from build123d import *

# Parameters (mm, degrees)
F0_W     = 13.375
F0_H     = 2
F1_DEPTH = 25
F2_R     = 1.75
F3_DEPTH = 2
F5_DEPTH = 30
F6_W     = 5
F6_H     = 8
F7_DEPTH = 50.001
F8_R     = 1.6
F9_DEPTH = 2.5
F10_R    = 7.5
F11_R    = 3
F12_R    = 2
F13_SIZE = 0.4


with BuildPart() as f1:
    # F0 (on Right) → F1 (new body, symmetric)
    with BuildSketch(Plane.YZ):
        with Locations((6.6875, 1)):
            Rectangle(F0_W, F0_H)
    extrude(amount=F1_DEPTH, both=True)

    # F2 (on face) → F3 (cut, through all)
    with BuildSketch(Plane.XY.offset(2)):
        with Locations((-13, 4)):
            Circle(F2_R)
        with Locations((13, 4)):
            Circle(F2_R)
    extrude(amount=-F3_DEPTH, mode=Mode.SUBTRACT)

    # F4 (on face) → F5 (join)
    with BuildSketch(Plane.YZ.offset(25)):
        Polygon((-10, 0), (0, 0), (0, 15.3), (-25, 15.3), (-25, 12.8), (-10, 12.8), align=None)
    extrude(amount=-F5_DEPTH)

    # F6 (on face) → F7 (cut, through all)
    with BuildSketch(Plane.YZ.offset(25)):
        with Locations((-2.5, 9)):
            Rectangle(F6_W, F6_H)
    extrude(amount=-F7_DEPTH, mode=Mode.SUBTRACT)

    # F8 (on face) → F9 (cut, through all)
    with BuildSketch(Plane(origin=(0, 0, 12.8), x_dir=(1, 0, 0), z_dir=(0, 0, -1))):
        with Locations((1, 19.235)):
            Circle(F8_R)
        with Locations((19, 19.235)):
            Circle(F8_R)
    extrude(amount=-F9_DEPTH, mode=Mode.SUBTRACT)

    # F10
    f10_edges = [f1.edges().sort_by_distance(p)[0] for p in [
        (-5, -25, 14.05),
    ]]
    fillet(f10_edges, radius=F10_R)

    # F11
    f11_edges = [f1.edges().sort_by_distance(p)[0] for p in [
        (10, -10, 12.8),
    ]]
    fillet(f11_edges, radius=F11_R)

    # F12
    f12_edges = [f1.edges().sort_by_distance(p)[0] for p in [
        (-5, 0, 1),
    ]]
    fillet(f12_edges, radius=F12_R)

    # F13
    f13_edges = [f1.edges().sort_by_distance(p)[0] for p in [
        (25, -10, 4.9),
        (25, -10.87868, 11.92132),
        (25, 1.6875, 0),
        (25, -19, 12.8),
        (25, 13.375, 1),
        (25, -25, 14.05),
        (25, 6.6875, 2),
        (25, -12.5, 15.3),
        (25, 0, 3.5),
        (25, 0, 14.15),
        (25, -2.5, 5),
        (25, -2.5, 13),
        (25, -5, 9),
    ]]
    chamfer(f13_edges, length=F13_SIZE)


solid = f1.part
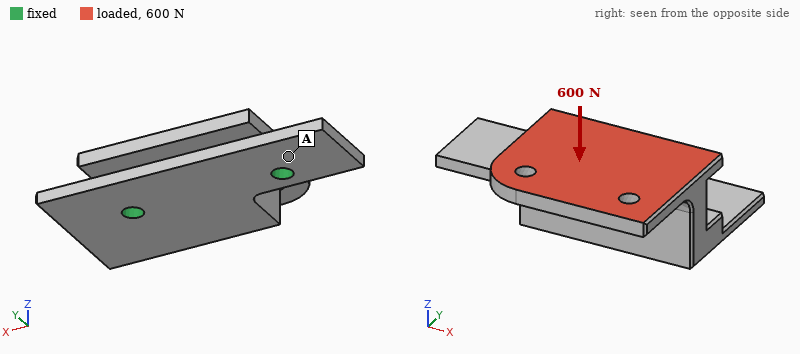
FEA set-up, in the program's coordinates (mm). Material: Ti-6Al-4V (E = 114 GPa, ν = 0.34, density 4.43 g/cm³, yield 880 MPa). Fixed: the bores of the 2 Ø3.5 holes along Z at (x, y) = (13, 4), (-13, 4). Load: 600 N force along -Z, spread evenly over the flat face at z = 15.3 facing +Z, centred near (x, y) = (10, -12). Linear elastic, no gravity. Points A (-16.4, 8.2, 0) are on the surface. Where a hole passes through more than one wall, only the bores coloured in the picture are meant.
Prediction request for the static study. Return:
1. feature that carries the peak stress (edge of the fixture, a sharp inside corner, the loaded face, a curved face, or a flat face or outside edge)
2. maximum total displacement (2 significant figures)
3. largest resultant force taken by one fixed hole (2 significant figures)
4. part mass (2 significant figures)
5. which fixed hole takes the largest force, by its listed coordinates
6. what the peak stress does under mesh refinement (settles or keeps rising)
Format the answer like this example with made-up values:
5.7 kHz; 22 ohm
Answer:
edge of the fixture; 0.63 mm; 550 N; 26 g; (13, 4); keeps rising
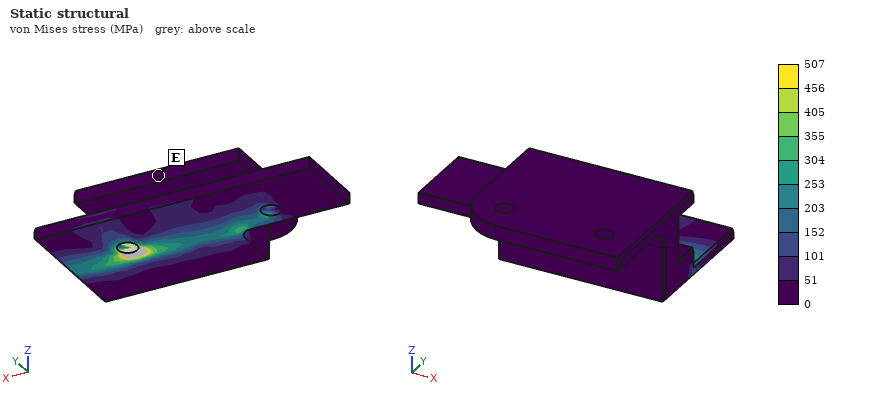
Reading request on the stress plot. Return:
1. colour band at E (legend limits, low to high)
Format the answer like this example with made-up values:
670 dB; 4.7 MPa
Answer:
0 to 51 MPa
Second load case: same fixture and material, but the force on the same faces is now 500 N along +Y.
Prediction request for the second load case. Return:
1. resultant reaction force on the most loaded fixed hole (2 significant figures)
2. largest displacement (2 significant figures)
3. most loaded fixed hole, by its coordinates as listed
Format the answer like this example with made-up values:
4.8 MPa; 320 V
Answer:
440 N; 0.53 mm; (13, 4)
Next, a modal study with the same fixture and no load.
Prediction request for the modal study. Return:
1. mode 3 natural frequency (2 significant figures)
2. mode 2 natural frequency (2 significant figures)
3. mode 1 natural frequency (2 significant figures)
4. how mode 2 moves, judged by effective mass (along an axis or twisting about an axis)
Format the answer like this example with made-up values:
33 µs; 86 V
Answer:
8200 Hz; 4300 Hz; 1500 Hz; along X
